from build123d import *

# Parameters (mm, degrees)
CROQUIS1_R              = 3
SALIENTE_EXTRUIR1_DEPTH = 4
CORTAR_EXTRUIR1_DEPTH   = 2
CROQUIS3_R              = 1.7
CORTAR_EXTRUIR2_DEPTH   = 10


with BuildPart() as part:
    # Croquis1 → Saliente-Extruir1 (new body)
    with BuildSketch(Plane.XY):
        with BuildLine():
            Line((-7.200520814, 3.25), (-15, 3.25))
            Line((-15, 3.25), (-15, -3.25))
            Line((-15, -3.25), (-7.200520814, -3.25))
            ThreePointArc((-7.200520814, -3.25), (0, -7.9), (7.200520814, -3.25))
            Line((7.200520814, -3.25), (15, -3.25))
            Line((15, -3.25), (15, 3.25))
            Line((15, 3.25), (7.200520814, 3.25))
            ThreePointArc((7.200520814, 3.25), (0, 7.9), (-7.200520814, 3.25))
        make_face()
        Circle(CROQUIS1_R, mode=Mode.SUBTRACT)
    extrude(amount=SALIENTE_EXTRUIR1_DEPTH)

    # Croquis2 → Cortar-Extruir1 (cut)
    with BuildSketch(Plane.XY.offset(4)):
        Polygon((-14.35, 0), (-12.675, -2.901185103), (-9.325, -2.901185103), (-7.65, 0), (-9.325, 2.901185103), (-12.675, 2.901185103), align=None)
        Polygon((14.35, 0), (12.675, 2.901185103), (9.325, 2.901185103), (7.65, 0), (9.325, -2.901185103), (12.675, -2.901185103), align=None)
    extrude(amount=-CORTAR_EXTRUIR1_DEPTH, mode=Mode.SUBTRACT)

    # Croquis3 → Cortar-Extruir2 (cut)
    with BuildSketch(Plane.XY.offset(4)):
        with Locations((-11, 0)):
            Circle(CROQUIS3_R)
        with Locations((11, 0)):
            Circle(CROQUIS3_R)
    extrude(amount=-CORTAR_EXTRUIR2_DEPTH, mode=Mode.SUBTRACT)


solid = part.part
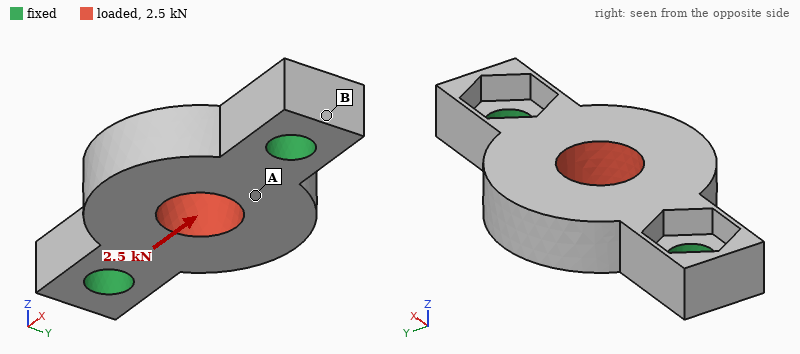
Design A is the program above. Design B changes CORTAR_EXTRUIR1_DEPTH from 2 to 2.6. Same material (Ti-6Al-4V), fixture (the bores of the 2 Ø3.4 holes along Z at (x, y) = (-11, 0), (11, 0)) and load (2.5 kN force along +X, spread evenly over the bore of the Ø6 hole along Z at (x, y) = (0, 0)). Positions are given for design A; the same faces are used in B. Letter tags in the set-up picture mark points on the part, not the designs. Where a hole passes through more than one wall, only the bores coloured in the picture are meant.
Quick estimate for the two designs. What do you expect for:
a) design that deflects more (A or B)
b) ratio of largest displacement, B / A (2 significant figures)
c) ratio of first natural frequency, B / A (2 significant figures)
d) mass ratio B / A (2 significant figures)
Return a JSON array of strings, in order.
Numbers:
["B", "1.2", "0.83", "0.97"]
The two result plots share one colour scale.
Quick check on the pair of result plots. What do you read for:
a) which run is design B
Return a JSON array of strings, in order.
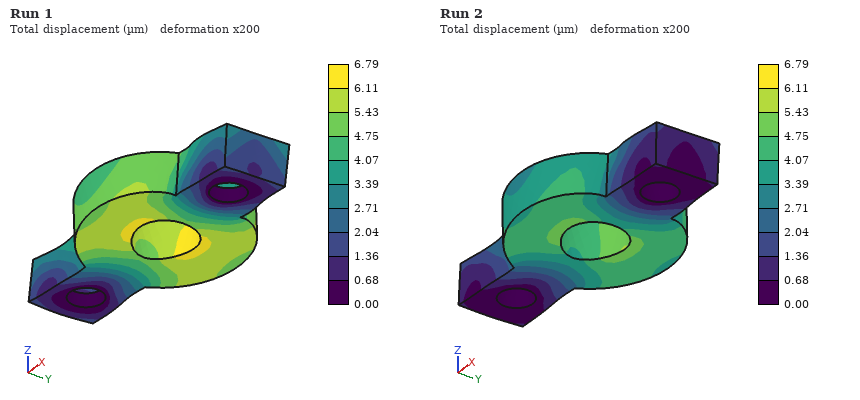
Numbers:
["Run 1"]
